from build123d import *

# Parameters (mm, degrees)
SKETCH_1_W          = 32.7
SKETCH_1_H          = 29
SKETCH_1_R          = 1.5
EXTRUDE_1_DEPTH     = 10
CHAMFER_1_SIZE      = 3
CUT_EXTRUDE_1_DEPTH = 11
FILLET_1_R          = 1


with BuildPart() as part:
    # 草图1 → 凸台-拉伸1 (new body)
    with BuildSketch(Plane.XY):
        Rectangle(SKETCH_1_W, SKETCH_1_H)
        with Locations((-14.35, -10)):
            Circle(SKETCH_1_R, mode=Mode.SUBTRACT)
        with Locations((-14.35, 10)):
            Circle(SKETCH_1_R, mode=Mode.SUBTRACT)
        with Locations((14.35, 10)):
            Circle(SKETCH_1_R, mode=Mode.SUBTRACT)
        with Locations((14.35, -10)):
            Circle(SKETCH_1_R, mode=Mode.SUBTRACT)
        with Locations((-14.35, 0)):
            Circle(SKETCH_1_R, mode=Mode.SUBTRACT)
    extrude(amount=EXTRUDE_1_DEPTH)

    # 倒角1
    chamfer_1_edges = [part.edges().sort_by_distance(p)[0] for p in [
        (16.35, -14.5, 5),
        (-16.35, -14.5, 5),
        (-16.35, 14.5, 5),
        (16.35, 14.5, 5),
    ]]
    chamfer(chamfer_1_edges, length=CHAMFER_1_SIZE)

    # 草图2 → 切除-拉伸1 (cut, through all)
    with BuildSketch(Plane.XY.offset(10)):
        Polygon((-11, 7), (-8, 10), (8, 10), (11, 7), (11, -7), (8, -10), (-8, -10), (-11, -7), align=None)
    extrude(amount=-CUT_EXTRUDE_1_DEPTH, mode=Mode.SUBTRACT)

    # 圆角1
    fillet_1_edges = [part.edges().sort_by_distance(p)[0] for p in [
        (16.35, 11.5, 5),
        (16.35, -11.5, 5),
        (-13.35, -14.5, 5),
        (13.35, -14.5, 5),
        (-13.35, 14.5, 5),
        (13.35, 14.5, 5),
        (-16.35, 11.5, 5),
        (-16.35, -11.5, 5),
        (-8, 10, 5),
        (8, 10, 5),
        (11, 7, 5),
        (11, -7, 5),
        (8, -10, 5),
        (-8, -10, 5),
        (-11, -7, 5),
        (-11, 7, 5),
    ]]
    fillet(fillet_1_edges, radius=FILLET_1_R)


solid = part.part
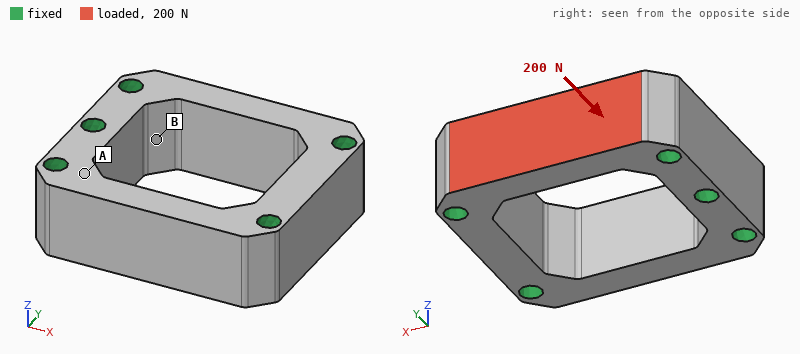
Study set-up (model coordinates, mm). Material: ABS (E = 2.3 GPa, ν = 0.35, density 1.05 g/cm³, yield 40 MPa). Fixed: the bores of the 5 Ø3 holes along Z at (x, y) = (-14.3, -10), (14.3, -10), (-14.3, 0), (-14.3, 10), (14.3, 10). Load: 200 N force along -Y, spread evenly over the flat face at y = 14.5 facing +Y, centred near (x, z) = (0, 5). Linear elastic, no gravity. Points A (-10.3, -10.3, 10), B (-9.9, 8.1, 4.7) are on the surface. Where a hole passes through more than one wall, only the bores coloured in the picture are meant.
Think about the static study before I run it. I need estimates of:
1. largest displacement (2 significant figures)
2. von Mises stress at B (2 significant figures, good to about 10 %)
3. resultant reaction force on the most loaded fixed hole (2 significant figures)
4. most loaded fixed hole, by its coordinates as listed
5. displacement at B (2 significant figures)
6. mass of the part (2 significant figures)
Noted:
51 µm
5.0 MPa
98 N
(14.3, 10)
9.7 µm
5.0 g
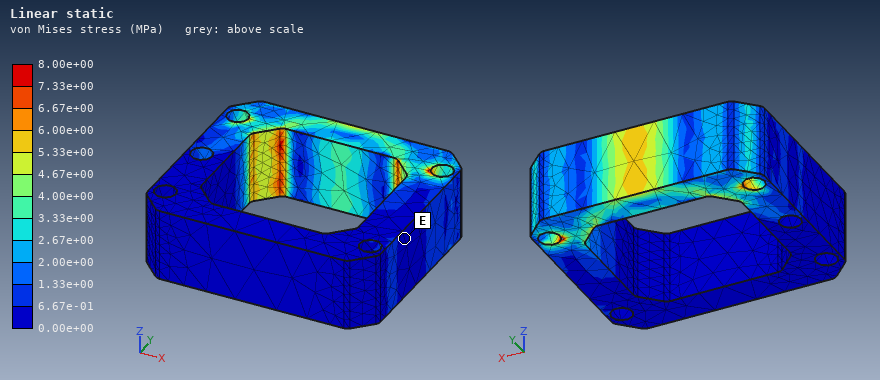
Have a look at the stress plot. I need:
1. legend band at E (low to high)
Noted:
0.00e+00 to 6.67e-01 MPa
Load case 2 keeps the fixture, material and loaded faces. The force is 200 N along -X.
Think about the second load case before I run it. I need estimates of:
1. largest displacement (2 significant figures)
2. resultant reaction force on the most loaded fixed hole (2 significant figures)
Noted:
8.8 µm
100 N
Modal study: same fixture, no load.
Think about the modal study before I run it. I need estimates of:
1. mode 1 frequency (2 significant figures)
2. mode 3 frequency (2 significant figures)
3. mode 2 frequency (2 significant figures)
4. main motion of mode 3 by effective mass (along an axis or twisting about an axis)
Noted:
10 kHz
13 kHz
10 kHz
along Z
